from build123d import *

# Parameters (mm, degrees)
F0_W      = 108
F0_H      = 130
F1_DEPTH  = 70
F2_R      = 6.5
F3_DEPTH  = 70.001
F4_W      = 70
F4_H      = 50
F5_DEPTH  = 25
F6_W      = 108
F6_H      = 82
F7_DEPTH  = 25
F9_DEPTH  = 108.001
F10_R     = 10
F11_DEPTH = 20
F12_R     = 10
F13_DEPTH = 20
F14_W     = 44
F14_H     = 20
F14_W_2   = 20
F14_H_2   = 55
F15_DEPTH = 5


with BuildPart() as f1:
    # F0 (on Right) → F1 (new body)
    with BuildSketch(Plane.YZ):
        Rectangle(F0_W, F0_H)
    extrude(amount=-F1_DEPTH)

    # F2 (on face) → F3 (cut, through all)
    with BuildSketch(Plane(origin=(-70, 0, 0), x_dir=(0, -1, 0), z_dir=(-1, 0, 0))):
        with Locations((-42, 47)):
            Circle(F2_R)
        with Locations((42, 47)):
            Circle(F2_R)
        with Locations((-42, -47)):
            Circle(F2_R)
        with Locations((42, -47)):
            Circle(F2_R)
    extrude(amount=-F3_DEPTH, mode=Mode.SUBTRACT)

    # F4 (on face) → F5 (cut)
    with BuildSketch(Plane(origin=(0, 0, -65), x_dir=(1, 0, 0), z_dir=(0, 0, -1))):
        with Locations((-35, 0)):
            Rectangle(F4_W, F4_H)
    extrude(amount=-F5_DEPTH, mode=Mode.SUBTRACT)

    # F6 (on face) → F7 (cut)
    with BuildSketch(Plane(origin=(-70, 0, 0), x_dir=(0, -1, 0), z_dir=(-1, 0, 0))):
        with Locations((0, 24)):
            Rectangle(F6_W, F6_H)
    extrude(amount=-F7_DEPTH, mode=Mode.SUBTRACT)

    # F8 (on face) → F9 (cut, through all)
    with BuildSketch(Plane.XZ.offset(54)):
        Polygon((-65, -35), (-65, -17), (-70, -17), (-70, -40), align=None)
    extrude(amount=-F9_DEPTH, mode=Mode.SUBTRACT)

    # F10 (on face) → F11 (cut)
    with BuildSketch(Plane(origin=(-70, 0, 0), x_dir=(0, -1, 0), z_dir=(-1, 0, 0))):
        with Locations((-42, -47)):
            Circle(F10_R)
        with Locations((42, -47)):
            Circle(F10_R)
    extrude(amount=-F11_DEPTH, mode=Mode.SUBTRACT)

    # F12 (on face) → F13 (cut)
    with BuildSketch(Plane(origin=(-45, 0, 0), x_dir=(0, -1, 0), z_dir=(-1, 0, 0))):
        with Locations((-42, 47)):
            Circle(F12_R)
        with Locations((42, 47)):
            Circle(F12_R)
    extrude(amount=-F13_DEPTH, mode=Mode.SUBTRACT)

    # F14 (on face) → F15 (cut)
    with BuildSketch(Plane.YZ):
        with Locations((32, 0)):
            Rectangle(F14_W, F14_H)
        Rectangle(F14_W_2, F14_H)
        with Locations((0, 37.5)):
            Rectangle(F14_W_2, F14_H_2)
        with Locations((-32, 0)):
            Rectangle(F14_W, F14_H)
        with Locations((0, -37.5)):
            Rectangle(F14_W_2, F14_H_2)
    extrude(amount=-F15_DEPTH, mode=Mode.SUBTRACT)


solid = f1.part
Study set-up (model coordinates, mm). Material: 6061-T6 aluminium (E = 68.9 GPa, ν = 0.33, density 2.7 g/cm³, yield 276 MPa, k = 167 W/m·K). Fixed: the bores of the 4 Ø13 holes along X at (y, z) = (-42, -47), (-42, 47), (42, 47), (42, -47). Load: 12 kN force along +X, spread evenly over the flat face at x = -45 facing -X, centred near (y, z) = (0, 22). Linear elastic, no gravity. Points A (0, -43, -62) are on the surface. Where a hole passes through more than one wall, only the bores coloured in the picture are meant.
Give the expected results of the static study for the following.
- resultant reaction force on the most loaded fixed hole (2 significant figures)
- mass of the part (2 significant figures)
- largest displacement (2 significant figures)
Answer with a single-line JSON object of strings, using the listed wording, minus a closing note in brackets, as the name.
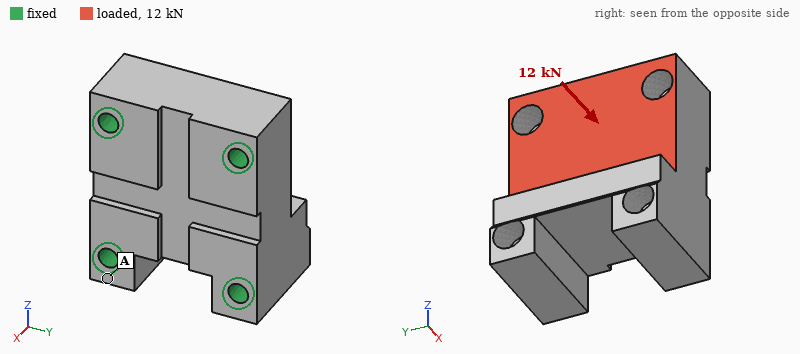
{"resultant reaction force on the most loaded fixed hole": "4.2 kN", "mass of the part": "1.6 kg", "largest displacement": "3.4 µm"}
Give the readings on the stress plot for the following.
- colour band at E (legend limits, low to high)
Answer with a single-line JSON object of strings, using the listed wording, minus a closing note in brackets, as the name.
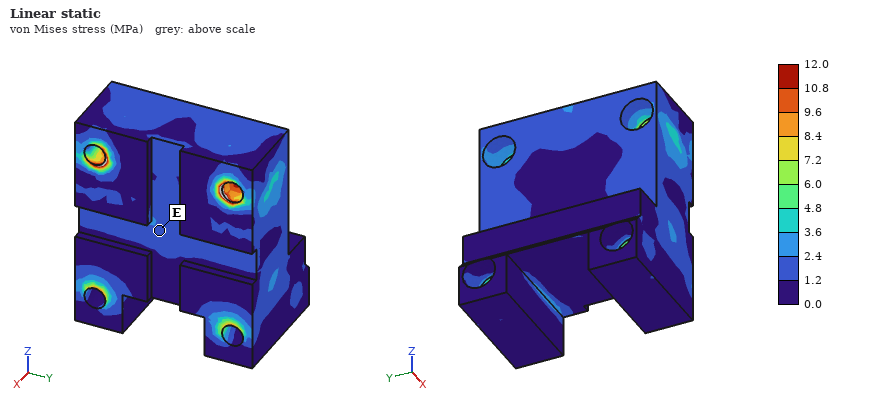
{"colour band at E": "1.2 to 2.4 MPa"}
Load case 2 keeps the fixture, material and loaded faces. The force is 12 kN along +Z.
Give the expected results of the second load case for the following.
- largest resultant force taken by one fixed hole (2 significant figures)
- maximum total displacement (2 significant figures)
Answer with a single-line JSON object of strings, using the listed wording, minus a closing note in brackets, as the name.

{"largest resultant force taken by one fixed hole": "4.1 kN", "maximum total displacement": "5.8 µm"}
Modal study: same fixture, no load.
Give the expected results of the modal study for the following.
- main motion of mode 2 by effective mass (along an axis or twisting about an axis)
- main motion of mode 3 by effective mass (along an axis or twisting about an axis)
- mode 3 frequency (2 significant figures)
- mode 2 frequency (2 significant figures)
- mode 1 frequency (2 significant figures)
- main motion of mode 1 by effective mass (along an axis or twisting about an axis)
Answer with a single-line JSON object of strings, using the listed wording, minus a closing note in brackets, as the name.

{"main motion of mode 2 by effective mass": "along Y", "main motion of mode 3 by effective mass": "along Z", "mode 3 frequency": "13 kHz", "mode 2 frequency": "12 kHz", "mode 1 frequency": "9800 Hz", "main motion of mode 1 by effective mass": "along X"}
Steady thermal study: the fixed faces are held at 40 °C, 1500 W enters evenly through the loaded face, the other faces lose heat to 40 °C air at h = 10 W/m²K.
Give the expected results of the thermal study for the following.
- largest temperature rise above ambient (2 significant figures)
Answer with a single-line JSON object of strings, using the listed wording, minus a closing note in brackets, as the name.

{"largest temperature rise above ambient": "59 K"}
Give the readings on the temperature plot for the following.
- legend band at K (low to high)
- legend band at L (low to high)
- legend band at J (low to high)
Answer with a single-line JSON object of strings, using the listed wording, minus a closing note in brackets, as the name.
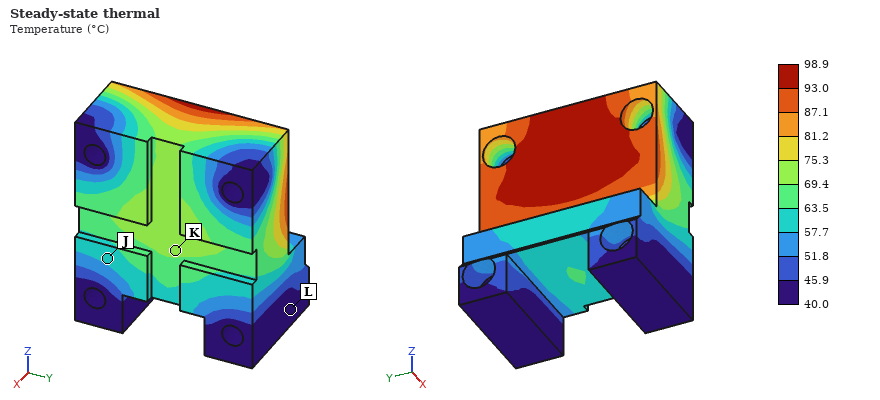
{"legend band at K": "69.4 to 75.3 °C", "legend band at L": "40.0 to 45.9 °C", "legend band at J": "57.7 to 63.5 °C"}
